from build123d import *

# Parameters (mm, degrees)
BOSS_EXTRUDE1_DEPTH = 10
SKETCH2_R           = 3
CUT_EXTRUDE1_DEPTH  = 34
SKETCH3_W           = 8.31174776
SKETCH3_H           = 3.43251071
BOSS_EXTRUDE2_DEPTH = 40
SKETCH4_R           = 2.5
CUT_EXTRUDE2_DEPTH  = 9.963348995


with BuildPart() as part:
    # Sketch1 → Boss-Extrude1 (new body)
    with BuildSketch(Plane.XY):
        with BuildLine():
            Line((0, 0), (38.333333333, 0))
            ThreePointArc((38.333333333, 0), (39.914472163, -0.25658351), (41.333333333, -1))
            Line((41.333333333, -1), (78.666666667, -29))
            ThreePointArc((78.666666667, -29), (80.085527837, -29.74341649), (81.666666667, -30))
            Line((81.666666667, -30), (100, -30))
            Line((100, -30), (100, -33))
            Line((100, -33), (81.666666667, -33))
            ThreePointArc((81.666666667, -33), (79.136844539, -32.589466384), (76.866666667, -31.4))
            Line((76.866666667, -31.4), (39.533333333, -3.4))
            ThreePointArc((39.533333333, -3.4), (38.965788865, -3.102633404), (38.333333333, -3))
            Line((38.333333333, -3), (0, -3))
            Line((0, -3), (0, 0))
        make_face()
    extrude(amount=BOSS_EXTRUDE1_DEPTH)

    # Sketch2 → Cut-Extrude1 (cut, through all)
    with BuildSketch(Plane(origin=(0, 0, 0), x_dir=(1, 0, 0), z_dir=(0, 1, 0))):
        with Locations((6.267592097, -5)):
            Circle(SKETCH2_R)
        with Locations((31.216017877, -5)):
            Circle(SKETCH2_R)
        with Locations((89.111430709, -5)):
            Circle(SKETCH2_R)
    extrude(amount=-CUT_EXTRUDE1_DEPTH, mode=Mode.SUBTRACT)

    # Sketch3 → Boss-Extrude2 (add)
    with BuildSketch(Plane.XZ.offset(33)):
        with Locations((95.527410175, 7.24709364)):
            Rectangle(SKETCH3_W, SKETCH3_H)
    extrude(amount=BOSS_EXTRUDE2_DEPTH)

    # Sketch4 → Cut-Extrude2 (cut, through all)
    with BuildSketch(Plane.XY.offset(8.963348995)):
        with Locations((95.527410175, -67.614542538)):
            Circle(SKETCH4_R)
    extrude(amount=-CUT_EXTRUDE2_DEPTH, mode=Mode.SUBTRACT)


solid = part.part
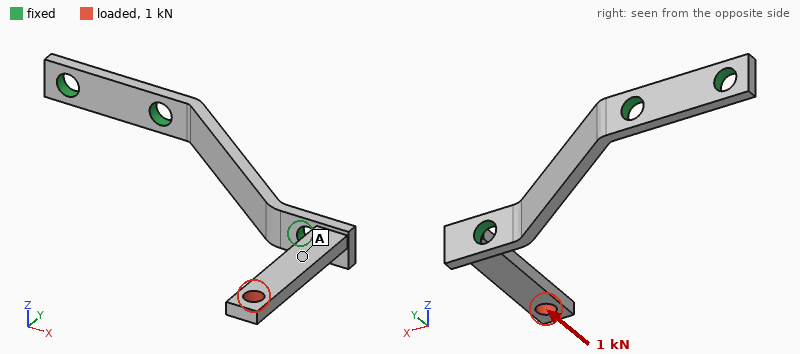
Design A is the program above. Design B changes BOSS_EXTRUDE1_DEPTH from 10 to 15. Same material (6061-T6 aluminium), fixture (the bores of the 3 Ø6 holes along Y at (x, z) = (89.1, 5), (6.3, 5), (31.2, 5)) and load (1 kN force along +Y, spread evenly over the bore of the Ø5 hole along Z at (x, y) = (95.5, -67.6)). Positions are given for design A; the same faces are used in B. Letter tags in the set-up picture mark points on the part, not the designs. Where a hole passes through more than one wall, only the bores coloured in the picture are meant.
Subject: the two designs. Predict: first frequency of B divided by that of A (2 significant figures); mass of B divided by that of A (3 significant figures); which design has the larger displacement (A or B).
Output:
1.0
1.40
A
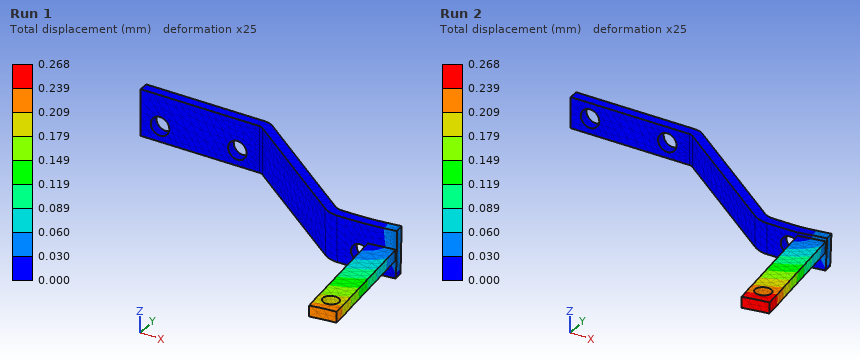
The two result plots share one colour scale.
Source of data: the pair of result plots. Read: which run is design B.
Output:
Run 1
